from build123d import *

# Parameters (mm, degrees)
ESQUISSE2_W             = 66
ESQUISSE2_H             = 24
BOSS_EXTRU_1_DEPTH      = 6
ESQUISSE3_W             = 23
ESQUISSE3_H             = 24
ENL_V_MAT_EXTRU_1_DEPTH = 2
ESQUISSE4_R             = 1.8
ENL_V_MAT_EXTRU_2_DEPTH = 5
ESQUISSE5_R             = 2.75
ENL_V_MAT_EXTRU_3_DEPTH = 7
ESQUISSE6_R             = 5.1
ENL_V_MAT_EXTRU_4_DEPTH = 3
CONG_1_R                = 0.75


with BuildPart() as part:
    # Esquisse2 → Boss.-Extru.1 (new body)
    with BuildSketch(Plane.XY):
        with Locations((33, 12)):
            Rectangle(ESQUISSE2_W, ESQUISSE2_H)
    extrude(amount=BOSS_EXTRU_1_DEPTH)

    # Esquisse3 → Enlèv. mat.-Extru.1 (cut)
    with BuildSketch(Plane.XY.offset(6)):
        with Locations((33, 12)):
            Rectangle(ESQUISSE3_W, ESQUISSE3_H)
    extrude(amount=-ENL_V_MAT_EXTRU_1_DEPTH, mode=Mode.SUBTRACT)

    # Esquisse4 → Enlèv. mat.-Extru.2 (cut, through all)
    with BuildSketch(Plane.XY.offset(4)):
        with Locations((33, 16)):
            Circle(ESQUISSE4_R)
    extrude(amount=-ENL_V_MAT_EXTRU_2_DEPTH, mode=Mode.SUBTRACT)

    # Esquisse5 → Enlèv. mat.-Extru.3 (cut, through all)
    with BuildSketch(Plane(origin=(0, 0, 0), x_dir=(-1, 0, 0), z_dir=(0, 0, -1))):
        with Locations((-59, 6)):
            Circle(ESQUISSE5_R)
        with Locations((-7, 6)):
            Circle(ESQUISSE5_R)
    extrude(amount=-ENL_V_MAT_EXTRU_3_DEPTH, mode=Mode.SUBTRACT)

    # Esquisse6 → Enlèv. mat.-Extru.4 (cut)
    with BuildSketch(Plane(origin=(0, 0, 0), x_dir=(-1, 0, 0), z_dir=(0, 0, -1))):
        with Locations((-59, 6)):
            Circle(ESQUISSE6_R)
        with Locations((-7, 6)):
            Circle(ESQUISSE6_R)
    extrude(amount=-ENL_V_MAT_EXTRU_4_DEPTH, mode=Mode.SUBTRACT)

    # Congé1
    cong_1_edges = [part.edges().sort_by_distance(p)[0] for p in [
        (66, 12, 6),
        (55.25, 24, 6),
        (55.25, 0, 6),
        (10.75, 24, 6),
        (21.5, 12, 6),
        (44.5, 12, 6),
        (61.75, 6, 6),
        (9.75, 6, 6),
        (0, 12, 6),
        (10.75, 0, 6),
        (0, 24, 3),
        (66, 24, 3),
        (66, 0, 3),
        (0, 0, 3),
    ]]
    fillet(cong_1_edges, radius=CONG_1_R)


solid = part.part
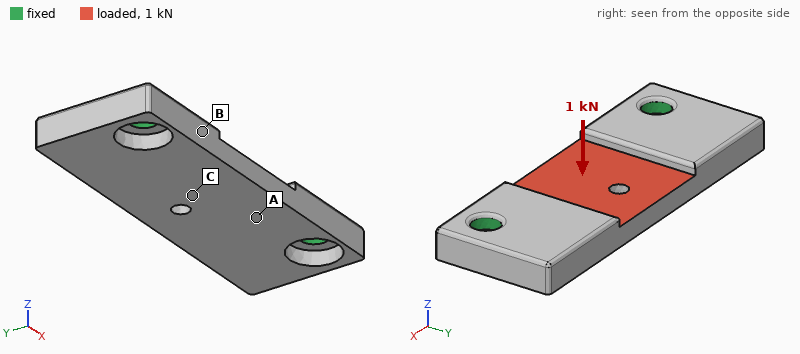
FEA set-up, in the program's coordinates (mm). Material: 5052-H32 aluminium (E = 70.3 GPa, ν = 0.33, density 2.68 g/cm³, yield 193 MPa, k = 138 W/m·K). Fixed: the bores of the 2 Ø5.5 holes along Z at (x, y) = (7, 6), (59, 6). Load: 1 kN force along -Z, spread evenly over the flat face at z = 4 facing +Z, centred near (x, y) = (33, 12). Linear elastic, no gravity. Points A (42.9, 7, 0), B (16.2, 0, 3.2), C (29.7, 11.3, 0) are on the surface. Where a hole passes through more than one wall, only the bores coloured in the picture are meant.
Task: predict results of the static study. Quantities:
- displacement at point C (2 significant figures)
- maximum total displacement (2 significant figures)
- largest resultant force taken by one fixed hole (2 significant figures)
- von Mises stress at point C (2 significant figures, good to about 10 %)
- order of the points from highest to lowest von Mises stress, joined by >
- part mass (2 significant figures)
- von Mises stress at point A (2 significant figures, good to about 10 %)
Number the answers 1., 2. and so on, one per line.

1. 0.069 mm
2. 0.11 mm
3. 1.1 kN
4. 58 MPa
5. C > A > B
6. 21 g
7. 34 MPa
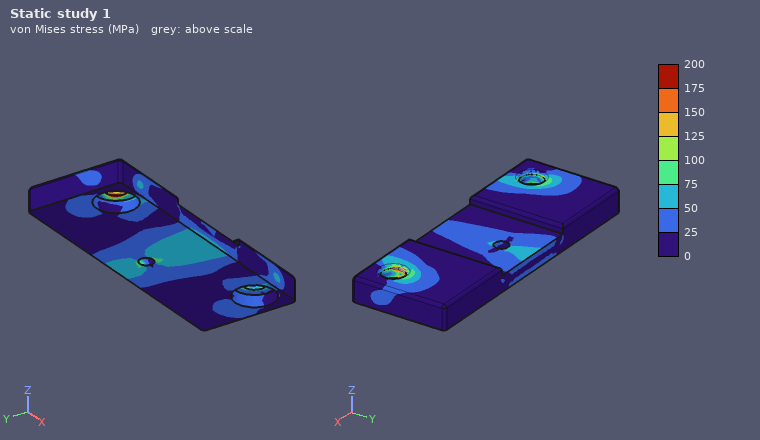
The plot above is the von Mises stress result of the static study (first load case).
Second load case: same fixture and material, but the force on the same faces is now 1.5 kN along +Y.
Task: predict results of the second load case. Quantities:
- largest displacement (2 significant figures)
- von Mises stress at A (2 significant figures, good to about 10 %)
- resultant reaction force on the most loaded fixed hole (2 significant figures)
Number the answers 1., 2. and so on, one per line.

1. 18 µm
2. 8.9 MPa
3. 820 N
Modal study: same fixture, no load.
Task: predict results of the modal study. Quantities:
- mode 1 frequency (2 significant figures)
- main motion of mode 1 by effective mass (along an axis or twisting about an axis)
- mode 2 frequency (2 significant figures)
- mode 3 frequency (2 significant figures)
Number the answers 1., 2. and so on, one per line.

1. 5700 Hz
2. along Z
3. 9700 Hz
4. 9900 Hz
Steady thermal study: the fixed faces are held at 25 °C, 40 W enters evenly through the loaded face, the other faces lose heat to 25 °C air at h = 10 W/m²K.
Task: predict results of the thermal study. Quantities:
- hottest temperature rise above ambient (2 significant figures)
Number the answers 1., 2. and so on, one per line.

1. 32 K
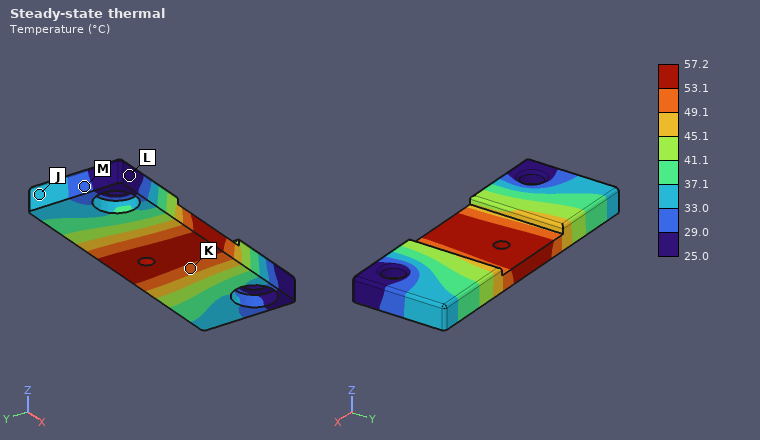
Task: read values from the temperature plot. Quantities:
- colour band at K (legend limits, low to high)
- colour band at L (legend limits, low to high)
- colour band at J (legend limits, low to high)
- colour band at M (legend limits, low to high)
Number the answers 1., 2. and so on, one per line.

1. 49.1 to 53.1 °C
2. 25.0 to 29.0 °C
3. 33.0 to 37.1 °C
4. 29.0 to 33.0 °C
